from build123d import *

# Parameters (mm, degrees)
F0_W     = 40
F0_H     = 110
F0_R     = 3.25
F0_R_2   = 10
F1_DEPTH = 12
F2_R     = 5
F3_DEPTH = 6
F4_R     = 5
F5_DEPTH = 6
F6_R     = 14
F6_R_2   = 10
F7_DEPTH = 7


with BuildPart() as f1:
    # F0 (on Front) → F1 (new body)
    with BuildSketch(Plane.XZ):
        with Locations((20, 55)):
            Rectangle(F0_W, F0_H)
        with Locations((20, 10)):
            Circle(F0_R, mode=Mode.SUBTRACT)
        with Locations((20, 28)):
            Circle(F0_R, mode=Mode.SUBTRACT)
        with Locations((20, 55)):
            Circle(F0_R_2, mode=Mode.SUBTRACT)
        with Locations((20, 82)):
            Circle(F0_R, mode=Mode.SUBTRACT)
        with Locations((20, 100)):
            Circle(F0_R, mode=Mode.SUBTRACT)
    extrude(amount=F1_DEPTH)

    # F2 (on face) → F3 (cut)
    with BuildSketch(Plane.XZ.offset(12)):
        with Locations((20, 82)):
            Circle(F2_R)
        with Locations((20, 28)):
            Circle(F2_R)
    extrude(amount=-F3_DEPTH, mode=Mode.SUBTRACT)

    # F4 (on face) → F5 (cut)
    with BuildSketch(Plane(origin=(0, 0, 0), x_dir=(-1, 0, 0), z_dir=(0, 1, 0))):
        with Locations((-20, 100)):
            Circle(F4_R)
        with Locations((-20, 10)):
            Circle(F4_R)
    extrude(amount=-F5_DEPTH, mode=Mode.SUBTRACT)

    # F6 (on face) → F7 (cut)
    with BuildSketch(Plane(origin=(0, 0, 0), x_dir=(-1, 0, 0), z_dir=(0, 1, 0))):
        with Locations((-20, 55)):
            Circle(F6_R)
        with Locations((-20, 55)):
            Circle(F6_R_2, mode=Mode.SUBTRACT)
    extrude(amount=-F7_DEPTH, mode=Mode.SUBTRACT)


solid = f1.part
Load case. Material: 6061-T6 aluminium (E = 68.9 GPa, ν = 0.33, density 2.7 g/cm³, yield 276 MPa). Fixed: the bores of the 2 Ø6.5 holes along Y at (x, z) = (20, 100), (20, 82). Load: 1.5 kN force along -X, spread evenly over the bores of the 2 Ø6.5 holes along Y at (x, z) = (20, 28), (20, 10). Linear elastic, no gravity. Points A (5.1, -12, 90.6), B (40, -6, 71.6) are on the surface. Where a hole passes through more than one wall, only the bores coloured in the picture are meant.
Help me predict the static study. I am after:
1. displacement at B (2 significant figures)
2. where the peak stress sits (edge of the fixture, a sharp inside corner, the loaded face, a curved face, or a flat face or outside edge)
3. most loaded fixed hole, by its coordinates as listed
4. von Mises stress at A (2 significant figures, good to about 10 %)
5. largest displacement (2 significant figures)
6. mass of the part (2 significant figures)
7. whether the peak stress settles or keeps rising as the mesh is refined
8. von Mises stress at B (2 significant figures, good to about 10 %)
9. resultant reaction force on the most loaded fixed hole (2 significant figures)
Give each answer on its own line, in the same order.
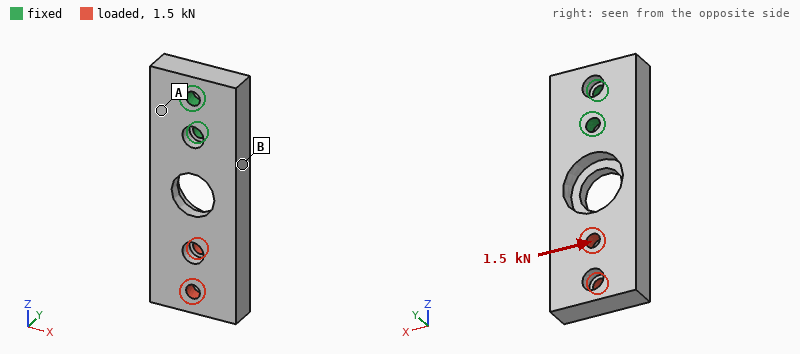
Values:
0.033 mm
edge of the fixture
(20, 82)
18 MPa
0.16 mm
120 g
keeps rising
41 MPa
4.8 kN
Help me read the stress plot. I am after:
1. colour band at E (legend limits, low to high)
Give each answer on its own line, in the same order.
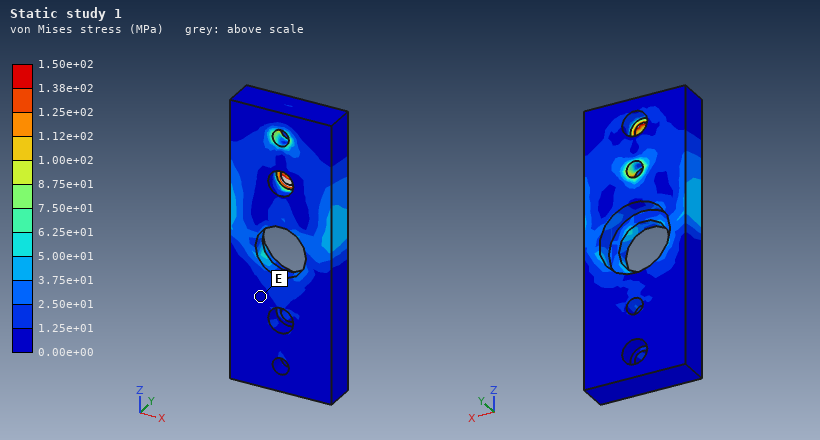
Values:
0.00e+00 to 1.25e+01 MPa
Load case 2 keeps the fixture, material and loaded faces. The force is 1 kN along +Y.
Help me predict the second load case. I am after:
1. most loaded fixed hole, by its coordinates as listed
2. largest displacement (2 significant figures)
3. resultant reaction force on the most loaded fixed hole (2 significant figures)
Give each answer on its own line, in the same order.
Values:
(20, 82)
0.63 mm
3.4 kN
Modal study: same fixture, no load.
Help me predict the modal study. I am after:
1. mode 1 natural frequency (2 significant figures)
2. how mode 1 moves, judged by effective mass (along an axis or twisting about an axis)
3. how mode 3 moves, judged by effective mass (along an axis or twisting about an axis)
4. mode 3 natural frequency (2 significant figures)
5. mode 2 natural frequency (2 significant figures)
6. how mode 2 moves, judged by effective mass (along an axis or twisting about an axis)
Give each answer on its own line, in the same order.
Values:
1100 Hz
along Y
twisting about Z
3500 Hz
2300 Hz
along X
